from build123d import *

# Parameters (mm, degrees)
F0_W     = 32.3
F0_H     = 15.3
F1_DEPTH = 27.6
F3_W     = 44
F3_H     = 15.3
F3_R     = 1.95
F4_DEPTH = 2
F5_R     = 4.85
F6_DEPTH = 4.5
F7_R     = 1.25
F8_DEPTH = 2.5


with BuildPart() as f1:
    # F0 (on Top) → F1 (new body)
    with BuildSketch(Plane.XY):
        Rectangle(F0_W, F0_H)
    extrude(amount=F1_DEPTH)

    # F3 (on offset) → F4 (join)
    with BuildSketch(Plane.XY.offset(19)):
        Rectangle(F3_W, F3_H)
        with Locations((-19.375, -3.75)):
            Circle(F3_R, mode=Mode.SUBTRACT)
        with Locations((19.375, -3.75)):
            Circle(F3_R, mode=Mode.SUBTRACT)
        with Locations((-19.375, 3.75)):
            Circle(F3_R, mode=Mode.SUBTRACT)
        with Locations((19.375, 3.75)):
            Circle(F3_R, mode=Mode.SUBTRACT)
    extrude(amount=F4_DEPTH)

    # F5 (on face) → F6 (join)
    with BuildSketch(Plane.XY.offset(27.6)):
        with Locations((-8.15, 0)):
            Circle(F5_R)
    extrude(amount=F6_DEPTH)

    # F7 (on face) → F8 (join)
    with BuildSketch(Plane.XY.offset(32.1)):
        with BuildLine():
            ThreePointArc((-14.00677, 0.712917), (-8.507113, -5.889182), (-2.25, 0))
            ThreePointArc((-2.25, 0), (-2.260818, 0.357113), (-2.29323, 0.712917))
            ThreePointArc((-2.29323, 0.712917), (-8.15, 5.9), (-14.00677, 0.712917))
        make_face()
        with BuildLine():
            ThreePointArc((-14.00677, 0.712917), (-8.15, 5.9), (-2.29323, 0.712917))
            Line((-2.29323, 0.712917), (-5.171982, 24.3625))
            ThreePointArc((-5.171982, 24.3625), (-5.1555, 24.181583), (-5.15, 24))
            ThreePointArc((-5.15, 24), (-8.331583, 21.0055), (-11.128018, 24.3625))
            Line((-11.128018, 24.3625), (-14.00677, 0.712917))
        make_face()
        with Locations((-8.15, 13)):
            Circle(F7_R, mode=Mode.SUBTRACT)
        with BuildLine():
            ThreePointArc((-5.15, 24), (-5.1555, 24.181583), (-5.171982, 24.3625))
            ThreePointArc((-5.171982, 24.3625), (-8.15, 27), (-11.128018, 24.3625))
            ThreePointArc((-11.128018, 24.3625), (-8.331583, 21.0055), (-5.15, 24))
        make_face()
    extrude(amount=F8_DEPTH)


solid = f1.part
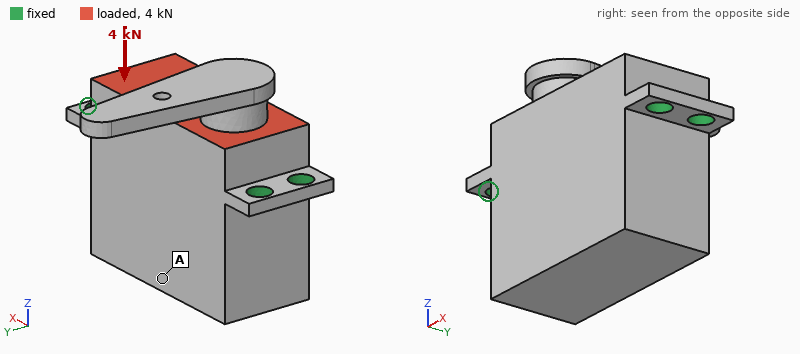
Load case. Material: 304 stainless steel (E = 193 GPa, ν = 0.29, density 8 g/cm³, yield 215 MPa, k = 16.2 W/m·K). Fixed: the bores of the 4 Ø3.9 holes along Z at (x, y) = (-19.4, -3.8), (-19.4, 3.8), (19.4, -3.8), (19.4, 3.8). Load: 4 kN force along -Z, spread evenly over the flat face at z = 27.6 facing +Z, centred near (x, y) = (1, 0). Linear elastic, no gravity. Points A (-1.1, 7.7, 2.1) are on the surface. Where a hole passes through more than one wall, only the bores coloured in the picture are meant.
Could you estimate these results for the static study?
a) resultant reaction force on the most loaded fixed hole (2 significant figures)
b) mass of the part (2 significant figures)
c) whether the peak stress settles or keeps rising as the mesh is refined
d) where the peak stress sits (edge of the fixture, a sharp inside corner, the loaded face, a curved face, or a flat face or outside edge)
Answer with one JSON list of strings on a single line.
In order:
["1.1 kN", "120 g", "keeps rising", "edge of the fixture"]
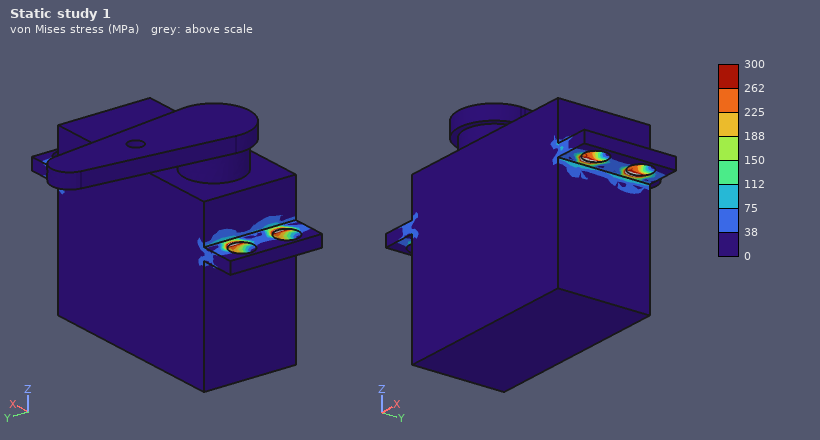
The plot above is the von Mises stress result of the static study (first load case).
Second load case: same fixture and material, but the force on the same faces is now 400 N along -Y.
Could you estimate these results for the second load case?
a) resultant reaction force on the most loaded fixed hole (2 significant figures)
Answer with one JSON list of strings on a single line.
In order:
["200 N"]
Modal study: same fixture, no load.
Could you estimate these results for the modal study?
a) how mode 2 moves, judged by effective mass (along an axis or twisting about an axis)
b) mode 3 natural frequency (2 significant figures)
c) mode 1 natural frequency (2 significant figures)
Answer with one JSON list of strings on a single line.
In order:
["along Y", "10 kHz", "4100 Hz"]
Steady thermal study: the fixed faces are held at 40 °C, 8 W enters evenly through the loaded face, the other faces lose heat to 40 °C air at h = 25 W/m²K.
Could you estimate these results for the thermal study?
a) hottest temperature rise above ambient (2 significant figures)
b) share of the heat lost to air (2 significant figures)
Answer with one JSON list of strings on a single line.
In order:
["31 K", "25 %"]
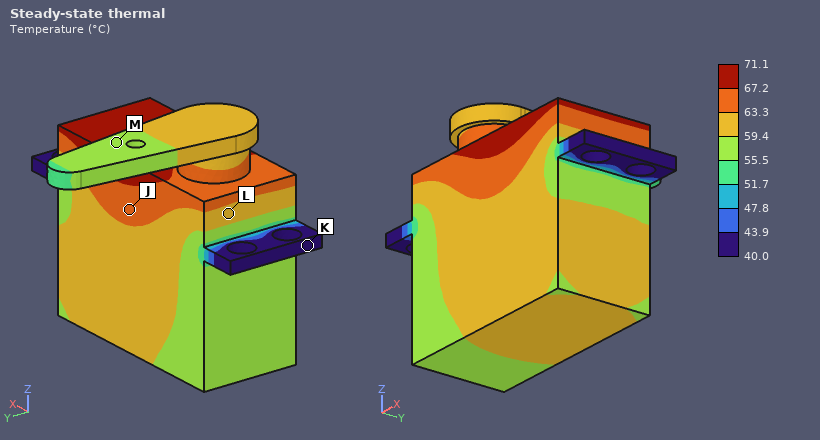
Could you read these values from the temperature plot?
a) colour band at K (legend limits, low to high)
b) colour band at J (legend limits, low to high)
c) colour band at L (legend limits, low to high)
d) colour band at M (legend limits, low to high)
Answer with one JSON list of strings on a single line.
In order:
["40.0 to 43.9 °C", "63.3 to 67.2 °C", "59.4 to 63.3 °C", "55.5 to 59.4 °C"]
